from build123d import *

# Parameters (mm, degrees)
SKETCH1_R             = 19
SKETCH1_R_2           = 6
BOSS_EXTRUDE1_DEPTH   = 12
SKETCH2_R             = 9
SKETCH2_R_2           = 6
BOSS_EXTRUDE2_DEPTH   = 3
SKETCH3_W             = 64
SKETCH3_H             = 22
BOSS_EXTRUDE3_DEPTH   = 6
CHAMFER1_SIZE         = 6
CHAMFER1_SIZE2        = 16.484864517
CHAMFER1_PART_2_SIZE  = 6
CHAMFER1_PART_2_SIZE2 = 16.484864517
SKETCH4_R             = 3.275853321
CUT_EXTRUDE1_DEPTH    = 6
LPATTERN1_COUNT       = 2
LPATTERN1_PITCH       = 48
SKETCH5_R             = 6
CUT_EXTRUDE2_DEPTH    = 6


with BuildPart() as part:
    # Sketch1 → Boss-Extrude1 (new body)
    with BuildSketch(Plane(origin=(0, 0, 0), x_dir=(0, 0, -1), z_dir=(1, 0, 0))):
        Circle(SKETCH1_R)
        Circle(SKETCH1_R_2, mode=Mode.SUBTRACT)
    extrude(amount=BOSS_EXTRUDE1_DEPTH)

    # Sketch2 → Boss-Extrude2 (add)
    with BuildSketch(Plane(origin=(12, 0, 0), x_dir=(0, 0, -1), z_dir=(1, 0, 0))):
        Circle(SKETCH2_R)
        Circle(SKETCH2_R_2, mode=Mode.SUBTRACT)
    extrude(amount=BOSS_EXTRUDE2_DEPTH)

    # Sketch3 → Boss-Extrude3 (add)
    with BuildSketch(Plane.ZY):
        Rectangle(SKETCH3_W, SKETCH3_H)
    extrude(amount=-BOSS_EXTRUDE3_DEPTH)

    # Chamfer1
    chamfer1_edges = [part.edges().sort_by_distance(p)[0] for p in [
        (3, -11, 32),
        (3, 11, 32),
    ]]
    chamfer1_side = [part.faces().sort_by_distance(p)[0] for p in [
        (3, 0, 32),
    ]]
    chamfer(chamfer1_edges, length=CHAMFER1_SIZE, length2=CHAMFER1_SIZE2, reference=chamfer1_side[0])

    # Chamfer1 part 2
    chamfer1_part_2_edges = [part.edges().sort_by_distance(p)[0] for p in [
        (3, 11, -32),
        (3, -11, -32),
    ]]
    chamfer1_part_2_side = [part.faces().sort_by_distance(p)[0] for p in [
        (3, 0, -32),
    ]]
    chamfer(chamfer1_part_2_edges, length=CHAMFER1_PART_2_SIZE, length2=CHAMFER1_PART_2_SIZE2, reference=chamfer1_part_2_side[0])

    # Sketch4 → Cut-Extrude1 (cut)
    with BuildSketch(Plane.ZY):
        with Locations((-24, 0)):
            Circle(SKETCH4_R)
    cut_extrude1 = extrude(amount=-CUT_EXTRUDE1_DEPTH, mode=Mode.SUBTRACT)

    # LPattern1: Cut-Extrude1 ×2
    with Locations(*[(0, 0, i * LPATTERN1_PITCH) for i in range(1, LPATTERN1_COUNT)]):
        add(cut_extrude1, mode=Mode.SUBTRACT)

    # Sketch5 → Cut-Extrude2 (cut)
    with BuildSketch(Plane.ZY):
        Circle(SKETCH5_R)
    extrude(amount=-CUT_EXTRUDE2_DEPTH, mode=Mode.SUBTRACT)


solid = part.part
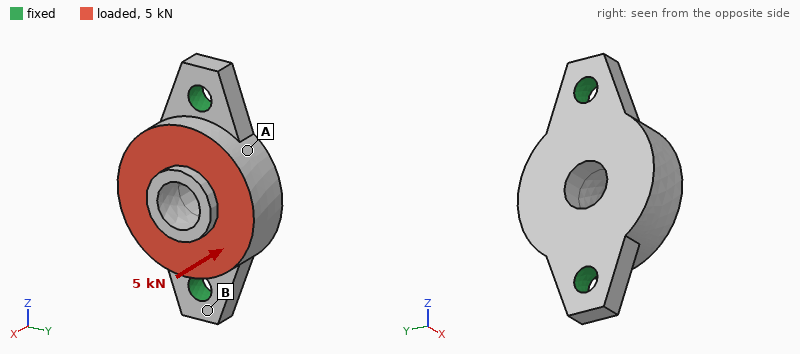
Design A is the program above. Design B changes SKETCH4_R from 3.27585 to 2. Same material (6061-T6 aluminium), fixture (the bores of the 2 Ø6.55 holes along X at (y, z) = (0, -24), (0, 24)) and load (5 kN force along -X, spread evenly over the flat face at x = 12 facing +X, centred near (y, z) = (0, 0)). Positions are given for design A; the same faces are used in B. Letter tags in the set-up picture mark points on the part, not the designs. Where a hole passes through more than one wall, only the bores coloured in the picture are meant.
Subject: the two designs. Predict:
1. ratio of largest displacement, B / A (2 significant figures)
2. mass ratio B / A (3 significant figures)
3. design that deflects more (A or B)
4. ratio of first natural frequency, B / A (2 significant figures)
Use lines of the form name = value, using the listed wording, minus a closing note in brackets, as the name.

ratio of largest displacement, B / A = 1.3
mass ratio B / A = 1.02
design that deflects more = B
ratio of first natural frequency, B / A = 0.83
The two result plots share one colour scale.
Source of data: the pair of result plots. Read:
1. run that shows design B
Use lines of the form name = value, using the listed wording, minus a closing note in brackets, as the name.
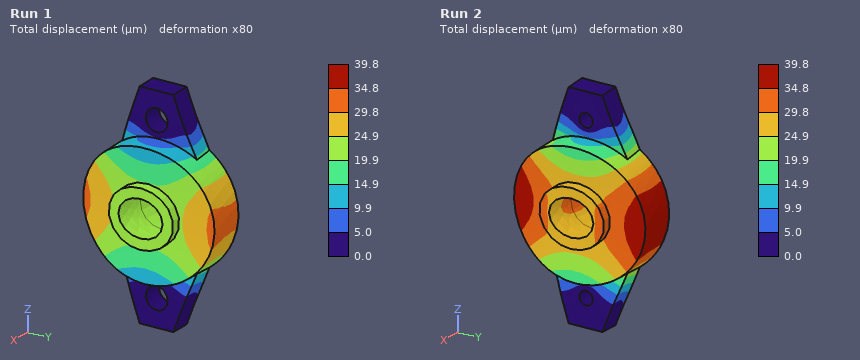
run that shows design B = Run 2
